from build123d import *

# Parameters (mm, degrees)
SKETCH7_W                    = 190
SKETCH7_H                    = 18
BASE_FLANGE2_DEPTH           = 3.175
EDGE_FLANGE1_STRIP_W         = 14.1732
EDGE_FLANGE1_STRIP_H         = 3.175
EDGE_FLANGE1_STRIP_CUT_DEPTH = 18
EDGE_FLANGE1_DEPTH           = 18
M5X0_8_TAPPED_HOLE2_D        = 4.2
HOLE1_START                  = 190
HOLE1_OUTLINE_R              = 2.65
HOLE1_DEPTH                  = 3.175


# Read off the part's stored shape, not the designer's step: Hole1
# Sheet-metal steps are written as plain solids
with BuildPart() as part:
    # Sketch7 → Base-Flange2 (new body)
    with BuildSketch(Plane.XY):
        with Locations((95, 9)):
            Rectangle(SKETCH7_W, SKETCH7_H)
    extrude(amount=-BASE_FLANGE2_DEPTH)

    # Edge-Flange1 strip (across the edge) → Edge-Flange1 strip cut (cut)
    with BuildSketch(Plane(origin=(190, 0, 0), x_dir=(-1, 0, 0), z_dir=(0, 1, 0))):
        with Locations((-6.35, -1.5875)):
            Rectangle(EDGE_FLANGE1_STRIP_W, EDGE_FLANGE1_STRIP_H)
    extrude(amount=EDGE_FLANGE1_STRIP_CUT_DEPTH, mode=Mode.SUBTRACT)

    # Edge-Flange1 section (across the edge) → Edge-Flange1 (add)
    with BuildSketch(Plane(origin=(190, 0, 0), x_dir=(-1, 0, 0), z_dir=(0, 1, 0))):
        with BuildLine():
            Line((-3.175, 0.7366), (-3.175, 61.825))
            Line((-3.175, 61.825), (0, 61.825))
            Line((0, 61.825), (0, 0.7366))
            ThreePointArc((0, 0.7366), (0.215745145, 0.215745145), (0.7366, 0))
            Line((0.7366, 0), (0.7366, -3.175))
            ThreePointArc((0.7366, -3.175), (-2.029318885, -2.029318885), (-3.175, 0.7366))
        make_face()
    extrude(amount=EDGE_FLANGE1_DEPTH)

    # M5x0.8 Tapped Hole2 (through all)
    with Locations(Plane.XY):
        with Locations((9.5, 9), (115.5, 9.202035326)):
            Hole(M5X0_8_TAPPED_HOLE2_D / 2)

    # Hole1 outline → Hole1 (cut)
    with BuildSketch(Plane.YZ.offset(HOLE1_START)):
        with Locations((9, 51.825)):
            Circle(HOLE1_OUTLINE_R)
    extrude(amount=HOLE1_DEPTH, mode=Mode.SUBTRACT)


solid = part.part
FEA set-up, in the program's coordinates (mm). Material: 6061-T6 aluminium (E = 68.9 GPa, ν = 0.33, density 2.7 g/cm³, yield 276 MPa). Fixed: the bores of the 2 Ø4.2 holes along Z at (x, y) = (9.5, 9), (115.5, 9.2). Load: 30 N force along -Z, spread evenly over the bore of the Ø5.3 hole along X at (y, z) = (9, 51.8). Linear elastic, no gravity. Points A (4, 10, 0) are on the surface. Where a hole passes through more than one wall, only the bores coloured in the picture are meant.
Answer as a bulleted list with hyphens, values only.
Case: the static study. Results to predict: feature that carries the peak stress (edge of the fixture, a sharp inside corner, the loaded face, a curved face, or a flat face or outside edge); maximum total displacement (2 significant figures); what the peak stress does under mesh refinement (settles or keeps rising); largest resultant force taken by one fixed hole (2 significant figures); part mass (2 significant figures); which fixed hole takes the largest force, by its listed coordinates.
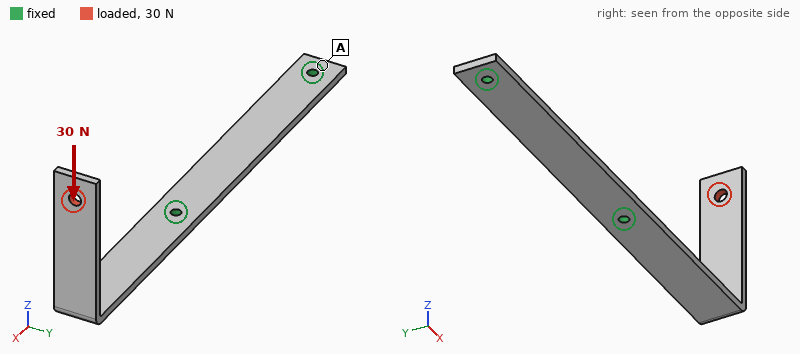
- edge of the fixture
- 2.1 mm
- keeps rising
- 30 N
- 39 g
- (115.5, 9.2)
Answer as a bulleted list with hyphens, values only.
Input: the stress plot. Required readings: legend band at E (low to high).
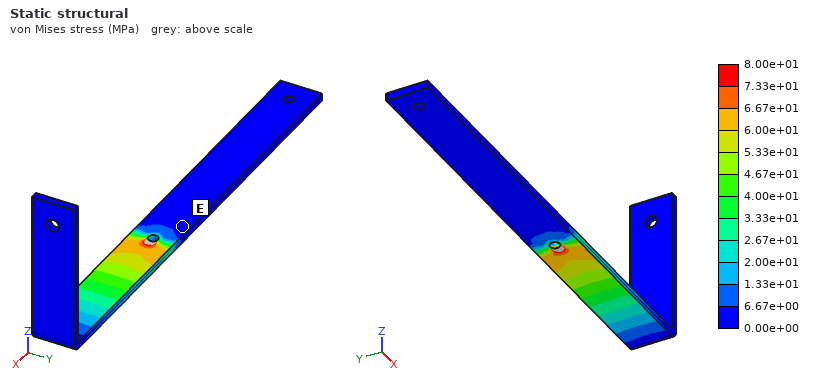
- 0.00e+00 to 6.67e+00 MPa
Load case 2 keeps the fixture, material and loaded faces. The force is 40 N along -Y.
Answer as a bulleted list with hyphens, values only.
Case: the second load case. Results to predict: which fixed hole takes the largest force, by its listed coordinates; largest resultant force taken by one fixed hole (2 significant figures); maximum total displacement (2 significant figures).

- (115.5, 9.2)
- 55 N
- 2.3 mm
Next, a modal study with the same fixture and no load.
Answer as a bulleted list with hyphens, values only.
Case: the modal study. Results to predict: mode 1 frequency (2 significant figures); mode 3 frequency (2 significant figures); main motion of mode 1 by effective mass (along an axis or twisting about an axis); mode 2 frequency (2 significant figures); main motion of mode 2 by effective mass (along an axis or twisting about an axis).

- 180 Hz
- 530 Hz
- along Z
- 340 Hz
- along Y
